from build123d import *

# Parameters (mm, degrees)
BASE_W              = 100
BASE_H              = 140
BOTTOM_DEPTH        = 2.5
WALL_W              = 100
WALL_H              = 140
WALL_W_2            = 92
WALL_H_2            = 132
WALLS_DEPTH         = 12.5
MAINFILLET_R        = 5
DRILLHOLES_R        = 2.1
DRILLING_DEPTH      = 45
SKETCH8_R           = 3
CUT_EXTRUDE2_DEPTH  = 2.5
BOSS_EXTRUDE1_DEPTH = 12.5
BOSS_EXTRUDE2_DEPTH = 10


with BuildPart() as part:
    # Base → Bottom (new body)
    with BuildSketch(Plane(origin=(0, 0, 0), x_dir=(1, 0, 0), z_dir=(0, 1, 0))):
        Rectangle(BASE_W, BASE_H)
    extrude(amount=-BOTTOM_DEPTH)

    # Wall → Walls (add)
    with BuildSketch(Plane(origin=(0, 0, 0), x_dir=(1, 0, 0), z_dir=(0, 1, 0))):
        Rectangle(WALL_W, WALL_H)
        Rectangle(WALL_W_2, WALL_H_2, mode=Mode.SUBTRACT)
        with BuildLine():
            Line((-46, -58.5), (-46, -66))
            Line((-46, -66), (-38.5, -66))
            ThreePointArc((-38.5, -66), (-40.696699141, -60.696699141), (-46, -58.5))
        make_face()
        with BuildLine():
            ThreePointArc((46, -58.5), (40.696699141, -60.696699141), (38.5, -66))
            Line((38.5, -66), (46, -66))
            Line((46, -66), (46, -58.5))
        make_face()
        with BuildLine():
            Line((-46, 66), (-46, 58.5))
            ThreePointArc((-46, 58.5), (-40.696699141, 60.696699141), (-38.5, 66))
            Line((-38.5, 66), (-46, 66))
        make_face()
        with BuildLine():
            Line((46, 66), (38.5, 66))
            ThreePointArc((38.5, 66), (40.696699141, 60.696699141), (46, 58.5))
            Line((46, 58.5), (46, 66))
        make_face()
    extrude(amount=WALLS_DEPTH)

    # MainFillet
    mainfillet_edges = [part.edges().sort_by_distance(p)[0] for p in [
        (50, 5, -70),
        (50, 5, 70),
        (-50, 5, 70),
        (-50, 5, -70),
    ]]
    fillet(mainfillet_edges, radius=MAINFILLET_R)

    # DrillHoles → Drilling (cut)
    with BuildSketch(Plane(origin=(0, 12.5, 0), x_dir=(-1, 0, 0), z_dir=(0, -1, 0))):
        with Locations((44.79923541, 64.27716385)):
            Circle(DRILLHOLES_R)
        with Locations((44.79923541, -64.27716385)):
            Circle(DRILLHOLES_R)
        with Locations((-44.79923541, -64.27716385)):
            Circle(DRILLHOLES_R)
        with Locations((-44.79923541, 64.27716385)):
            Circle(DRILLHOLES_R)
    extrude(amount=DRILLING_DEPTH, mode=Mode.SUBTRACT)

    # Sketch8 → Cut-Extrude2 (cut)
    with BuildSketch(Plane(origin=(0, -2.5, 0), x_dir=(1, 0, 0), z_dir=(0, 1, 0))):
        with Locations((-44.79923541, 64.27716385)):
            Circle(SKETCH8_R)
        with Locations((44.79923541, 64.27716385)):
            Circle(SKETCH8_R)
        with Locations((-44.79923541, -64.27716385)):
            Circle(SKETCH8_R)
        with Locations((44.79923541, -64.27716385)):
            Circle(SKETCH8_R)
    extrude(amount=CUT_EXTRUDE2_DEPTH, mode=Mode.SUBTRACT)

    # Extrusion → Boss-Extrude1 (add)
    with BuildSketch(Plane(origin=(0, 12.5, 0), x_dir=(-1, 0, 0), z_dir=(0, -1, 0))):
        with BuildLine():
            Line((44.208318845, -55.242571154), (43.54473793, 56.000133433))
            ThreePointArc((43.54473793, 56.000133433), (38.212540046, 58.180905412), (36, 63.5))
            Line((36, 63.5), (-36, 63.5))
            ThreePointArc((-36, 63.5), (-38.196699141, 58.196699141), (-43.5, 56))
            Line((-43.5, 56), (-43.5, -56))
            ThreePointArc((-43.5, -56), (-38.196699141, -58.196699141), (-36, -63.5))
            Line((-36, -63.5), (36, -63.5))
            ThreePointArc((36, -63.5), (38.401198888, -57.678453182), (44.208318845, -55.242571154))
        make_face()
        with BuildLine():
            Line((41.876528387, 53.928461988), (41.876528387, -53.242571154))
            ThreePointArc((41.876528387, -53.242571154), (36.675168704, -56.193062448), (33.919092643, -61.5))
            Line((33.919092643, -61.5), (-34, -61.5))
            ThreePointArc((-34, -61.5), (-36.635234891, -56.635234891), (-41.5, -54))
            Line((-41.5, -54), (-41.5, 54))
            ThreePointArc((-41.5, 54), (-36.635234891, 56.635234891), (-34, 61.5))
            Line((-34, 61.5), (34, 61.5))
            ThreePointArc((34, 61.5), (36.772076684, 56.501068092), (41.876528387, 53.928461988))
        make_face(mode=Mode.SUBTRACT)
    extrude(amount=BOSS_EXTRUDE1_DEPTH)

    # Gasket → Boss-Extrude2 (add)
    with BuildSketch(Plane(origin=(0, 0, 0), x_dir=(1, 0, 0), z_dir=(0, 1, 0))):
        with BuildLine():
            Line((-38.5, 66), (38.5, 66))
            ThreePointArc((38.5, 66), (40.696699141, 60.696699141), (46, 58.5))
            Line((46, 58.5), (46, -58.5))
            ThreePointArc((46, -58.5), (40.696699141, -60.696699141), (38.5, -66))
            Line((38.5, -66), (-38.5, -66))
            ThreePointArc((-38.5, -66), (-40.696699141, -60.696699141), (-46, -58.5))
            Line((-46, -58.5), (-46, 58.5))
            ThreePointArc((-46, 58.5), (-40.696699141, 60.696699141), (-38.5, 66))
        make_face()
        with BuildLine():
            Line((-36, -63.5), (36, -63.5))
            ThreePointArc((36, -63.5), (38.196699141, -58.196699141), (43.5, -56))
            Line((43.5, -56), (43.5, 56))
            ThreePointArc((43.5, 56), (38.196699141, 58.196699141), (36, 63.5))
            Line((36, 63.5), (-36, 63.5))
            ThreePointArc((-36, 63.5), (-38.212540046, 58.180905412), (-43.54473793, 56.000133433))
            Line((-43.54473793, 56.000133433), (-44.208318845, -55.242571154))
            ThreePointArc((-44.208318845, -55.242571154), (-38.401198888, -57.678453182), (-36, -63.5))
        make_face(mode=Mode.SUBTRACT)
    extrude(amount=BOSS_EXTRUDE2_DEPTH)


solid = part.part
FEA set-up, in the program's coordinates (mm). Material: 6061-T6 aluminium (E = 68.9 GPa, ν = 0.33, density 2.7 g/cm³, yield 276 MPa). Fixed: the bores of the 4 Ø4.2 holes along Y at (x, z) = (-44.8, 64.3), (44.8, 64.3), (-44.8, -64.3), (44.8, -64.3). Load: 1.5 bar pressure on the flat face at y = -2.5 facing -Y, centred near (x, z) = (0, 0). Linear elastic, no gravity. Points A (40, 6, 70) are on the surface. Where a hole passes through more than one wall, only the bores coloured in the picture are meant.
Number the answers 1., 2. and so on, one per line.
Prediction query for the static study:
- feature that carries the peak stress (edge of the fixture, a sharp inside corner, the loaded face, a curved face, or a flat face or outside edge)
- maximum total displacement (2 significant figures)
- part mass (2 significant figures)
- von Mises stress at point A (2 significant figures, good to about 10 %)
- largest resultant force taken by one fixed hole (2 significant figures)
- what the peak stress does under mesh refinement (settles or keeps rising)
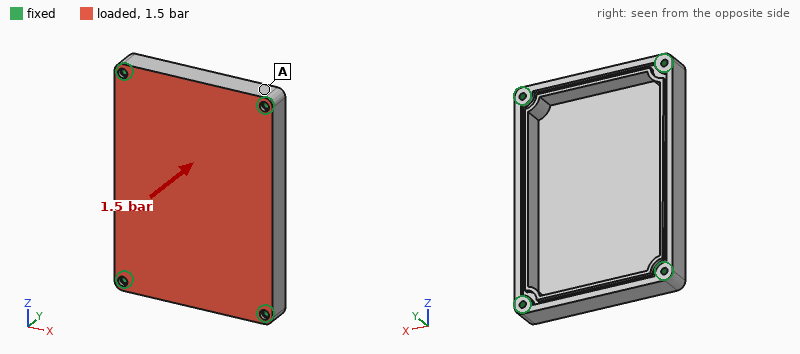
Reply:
1. edge of the fixture
2. 0.24 mm
3. 220 g
4. 7.7 MPa
5. 680 N
6. keeps rising
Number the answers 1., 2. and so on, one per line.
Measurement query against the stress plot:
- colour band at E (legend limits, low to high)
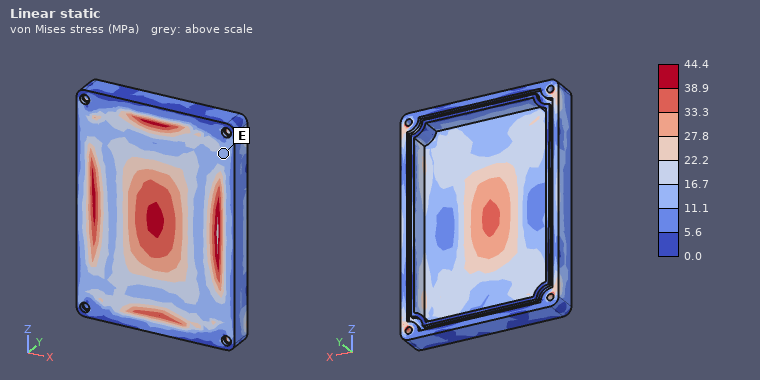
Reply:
1. 11.1 to 16.7 MPa
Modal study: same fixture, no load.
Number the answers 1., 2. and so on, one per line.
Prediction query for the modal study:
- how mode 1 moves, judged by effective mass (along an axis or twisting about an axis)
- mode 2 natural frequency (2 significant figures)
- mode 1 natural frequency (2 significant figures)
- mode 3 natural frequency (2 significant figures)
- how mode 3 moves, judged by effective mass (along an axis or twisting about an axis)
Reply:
1. along Y
2. 3300 Hz
3. 1900 Hz
4. 3600 Hz
5. twisting about Z
